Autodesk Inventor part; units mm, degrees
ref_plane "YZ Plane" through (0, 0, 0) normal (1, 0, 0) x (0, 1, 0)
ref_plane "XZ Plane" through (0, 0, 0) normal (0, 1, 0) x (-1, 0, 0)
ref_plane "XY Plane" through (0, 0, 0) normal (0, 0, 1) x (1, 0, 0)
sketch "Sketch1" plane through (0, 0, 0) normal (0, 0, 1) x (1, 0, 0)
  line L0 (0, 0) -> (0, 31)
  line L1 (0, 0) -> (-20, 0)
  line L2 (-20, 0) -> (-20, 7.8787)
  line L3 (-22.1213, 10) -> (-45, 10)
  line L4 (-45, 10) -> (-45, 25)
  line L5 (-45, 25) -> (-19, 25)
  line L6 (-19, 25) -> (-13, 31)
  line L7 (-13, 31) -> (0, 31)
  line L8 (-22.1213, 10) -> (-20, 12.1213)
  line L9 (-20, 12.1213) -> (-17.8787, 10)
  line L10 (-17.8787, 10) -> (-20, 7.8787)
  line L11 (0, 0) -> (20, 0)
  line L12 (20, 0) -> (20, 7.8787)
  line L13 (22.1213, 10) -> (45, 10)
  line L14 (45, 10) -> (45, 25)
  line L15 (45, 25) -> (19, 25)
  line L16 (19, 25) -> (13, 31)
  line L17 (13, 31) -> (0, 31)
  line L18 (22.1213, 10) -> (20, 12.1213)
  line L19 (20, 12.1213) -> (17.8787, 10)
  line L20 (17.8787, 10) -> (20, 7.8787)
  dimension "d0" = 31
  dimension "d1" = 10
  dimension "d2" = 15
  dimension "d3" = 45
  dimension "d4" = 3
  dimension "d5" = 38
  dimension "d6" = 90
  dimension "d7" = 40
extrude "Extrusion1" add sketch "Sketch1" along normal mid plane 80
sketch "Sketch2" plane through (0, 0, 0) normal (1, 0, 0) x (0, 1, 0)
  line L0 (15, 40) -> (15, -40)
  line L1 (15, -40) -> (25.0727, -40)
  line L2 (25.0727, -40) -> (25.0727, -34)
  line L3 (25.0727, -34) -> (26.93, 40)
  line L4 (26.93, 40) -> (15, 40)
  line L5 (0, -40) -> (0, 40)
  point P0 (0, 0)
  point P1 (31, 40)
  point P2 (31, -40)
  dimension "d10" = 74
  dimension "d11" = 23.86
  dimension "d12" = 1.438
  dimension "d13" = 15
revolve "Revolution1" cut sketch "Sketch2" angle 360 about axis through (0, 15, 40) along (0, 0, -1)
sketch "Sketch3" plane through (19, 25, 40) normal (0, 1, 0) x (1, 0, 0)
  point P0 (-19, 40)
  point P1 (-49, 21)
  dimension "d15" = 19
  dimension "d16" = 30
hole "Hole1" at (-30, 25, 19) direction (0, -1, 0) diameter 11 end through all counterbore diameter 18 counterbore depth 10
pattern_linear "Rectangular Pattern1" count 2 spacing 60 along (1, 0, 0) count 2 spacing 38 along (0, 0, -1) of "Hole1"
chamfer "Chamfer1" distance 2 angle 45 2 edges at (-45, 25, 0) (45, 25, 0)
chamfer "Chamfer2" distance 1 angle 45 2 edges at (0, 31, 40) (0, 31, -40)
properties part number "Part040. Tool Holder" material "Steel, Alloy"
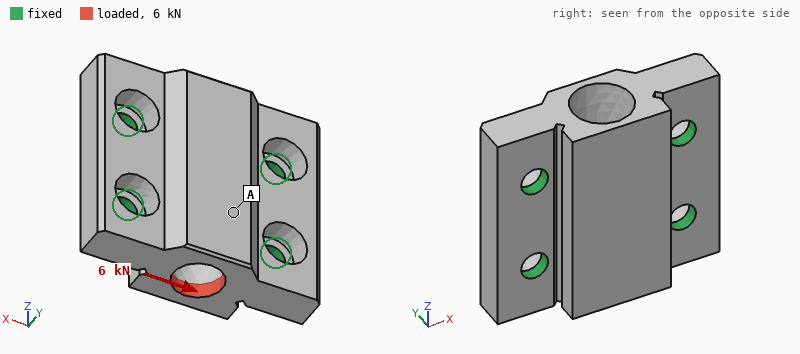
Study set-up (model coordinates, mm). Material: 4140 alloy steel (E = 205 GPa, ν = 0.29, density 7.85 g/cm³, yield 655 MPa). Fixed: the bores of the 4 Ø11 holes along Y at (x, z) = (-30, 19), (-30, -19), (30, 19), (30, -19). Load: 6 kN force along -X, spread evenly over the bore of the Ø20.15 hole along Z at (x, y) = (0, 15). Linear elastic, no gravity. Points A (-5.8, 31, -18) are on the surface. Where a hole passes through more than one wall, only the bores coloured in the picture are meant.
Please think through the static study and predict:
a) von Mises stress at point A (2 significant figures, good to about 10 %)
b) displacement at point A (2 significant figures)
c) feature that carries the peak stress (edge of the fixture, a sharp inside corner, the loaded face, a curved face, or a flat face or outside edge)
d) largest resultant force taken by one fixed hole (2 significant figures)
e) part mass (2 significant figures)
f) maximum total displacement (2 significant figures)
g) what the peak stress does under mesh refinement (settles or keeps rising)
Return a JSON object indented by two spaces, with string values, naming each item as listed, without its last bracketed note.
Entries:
{
  "von Mises stress at point A": "4.6 MPa",
  "displacement at point A": "1.0 µm",
  "feature that carries the peak stress": "edge of the fixture",
  "largest resultant force taken by one fixed hole": "3.0 kN",
  "part mass": "880 g",
  "maximum total displacement": "4.0 µm",
  "what the peak stress does under mesh refinement": "keeps rising"
}
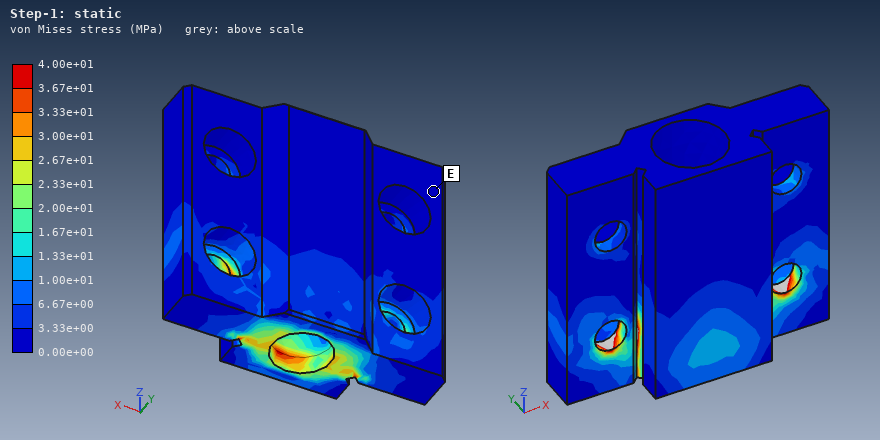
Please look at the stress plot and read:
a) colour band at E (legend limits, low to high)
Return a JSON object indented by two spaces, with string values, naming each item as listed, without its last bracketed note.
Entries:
{
  "colour band at E": "0.00e+00 to 3.33e+00 MPa"
}
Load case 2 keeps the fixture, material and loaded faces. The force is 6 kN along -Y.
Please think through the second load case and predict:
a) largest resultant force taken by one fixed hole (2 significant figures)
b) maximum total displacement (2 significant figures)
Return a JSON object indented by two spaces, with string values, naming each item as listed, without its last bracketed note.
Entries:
{
  "largest resultant force taken by one fixed hole": "4.3 kN",
  "maximum total displacement": "14 µm"
}
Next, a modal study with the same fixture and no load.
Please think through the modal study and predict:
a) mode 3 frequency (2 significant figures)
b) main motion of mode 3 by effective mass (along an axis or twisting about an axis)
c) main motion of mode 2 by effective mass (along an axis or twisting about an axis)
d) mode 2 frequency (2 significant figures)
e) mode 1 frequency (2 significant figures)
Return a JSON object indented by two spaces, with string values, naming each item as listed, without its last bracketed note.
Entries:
{
  "mode 3 frequency": "14 kHz",
  "main motion of mode 3 by effective mass": "along X",
  "main motion of mode 2 by effective mass": "along Y",
  "mode 2 frequency": "12 kHz",
  "mode 1 frequency": "9800 Hz"
}
